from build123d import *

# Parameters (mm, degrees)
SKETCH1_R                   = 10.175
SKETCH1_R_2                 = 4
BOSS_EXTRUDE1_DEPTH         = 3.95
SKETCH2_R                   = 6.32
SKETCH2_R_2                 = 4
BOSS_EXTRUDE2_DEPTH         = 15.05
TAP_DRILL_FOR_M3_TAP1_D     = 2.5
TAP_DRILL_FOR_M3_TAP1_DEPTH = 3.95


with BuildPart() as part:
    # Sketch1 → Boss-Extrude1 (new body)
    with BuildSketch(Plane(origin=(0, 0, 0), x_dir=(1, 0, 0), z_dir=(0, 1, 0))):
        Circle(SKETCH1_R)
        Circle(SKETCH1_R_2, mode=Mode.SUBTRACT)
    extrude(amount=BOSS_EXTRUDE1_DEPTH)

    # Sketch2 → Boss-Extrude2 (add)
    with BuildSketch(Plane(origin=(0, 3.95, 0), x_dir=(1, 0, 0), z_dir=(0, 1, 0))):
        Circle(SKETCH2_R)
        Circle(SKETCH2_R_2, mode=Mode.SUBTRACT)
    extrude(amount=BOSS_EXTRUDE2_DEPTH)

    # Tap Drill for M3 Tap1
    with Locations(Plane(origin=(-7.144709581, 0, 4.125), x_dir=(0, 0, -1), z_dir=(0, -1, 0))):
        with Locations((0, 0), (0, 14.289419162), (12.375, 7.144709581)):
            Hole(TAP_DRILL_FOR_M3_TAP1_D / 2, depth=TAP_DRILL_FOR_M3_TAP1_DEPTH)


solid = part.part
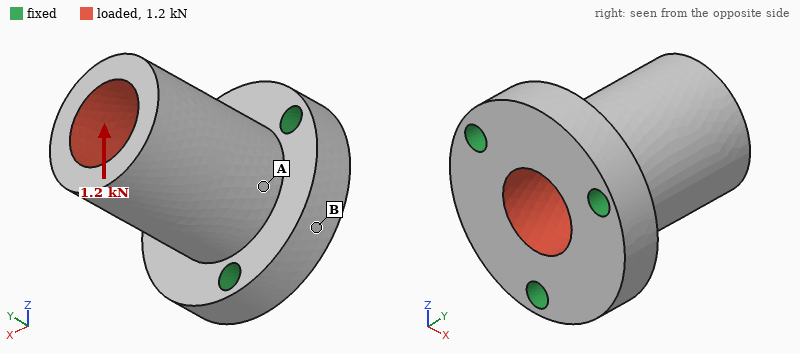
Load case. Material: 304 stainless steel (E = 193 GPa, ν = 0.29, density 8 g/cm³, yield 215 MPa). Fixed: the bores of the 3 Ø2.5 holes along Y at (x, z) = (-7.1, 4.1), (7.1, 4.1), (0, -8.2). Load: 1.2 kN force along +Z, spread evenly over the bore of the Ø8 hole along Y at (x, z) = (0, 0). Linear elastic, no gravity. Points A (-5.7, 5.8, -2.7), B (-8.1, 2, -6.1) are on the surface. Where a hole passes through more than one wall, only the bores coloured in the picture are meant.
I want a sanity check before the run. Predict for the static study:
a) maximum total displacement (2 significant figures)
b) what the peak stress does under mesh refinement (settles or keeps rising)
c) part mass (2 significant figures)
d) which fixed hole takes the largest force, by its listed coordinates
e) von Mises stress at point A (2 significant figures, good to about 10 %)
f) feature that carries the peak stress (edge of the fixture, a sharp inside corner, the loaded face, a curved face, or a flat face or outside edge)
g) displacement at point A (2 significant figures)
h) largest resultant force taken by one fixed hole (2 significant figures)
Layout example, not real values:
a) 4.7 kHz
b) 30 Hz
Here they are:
a) 8.6 µm
b) keeps rising
c) 17 g
d) (0, -8.2)
e) 26 MPa
f) a sharp inside corner
g) 1.8 µm
h) 810 N
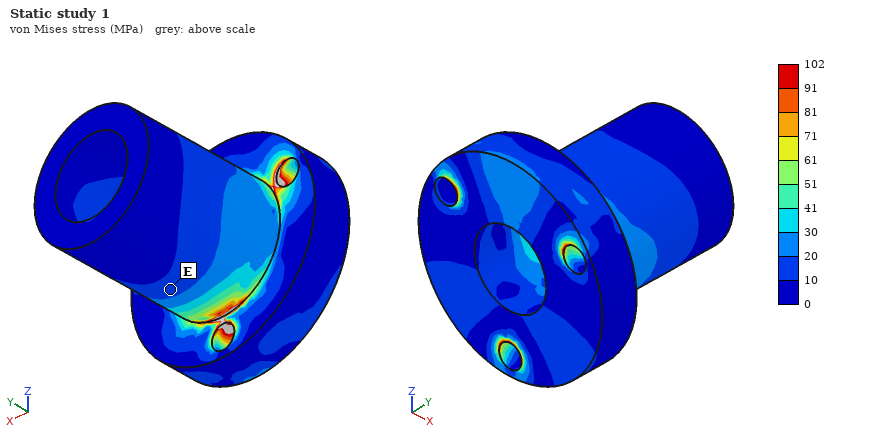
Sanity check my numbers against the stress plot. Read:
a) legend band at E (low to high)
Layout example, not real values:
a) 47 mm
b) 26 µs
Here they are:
a) 10 to 20 MPa
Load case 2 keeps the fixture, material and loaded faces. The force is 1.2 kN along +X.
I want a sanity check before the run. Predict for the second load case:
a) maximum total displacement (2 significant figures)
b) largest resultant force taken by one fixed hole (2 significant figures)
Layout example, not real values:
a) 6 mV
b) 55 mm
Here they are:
a) 8.6 µm
b) 730 N
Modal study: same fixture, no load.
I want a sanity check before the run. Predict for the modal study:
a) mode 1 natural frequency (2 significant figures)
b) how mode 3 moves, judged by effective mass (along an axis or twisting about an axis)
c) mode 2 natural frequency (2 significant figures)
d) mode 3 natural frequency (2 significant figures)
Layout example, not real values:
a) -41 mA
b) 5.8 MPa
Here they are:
a) 21 kHz
b) twisting about Y
c) 21 kHz
d) 46 kHz
